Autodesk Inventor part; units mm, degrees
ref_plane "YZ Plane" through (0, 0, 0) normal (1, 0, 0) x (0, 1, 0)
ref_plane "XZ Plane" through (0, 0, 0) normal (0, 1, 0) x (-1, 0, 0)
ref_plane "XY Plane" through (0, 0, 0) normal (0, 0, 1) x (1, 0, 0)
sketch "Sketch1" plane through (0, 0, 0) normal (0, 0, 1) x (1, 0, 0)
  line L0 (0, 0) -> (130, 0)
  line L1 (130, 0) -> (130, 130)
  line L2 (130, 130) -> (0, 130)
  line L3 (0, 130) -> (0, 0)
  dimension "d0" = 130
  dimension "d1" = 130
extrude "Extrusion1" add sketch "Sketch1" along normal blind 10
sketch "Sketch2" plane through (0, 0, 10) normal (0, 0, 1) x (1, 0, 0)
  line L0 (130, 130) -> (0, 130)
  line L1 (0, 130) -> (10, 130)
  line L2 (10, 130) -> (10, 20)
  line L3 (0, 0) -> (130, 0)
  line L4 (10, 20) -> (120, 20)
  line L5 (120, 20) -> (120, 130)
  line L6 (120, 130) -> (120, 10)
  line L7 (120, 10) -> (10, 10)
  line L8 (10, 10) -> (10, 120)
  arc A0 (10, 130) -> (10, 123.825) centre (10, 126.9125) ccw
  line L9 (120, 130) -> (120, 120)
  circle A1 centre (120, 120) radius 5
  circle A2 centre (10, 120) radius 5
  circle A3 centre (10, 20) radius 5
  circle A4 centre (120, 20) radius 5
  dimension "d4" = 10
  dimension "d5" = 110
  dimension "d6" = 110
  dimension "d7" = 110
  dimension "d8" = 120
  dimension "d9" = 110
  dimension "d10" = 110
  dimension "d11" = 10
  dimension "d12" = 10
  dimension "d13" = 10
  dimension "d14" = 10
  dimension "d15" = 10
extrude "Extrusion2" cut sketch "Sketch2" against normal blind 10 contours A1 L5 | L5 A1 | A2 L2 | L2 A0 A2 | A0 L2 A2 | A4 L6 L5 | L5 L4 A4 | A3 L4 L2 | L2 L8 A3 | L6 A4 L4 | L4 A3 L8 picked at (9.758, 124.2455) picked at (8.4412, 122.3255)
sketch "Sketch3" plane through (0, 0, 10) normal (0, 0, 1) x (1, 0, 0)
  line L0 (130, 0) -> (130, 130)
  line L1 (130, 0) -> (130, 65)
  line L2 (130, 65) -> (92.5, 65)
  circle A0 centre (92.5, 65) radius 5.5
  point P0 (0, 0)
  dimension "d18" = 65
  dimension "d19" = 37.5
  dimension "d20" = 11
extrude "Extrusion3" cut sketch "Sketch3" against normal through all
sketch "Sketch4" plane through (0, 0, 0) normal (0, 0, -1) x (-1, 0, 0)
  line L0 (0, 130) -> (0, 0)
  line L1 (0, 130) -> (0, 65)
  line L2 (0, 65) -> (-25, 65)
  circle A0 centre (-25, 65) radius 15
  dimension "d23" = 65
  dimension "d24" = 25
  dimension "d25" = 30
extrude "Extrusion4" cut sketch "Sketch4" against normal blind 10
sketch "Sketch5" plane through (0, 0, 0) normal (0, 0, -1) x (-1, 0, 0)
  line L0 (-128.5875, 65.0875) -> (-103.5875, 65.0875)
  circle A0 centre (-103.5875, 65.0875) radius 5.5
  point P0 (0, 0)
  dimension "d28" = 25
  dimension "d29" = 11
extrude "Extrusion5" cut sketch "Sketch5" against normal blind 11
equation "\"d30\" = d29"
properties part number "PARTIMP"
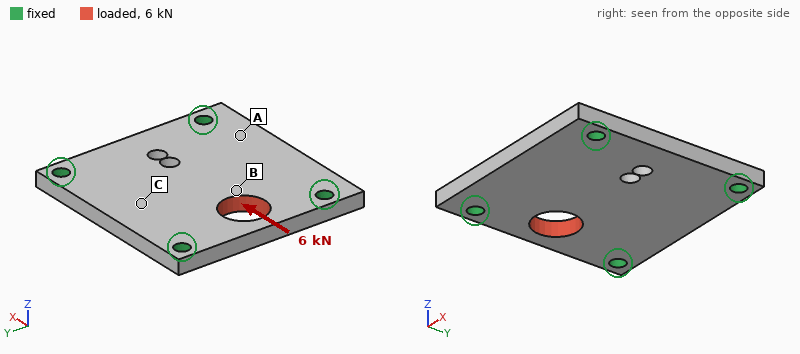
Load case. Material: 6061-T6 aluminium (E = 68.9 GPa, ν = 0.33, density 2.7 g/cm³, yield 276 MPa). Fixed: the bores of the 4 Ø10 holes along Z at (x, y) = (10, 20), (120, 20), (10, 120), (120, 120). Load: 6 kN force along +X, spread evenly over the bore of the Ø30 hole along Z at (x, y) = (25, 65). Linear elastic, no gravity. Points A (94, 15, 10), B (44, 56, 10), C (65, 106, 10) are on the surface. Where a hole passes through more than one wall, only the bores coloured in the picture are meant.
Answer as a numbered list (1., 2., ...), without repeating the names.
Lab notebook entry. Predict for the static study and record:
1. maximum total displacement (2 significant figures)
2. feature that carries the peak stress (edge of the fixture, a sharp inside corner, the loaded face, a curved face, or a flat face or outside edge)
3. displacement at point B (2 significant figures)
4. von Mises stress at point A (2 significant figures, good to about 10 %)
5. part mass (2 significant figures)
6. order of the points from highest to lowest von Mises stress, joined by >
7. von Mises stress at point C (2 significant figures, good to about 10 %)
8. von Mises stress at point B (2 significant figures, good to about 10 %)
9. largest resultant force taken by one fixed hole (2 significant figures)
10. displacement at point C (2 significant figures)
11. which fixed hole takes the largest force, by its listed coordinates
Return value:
1. 15 µm
2. edge of the fixture
3. 5.3 µm
4. 2.5 MPa
5. 420 g
6. B > C > A
7. 4.1 MPa
8. 7.3 MPa
9. 2.0 kN
10. 3.0 µm
11. (10, 20)
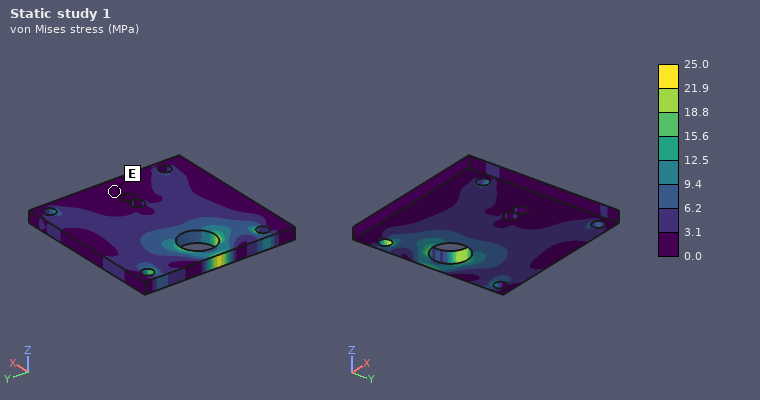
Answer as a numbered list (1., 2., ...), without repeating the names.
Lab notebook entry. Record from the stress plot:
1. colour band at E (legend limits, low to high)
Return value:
1. 0.0 to 3.1 MPa
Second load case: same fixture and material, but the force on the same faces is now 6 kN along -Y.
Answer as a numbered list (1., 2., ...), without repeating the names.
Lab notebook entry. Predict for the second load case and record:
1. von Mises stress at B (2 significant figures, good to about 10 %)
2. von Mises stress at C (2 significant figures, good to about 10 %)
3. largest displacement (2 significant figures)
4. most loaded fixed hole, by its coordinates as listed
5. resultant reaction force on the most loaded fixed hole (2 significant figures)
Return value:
1. 3.6 MPa
2. 2.2 MPa
3. 6.0 µm
4. (10, 20)
5. 2.6 kN
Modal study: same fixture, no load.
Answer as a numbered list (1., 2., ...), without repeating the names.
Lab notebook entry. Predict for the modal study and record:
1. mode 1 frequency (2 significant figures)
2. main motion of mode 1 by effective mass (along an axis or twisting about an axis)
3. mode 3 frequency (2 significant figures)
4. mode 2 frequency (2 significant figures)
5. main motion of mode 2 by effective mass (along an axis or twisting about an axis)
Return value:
1. 3100 Hz
2. along Z
3. 5400 Hz
4. 4600 Hz
5. twisting about X
